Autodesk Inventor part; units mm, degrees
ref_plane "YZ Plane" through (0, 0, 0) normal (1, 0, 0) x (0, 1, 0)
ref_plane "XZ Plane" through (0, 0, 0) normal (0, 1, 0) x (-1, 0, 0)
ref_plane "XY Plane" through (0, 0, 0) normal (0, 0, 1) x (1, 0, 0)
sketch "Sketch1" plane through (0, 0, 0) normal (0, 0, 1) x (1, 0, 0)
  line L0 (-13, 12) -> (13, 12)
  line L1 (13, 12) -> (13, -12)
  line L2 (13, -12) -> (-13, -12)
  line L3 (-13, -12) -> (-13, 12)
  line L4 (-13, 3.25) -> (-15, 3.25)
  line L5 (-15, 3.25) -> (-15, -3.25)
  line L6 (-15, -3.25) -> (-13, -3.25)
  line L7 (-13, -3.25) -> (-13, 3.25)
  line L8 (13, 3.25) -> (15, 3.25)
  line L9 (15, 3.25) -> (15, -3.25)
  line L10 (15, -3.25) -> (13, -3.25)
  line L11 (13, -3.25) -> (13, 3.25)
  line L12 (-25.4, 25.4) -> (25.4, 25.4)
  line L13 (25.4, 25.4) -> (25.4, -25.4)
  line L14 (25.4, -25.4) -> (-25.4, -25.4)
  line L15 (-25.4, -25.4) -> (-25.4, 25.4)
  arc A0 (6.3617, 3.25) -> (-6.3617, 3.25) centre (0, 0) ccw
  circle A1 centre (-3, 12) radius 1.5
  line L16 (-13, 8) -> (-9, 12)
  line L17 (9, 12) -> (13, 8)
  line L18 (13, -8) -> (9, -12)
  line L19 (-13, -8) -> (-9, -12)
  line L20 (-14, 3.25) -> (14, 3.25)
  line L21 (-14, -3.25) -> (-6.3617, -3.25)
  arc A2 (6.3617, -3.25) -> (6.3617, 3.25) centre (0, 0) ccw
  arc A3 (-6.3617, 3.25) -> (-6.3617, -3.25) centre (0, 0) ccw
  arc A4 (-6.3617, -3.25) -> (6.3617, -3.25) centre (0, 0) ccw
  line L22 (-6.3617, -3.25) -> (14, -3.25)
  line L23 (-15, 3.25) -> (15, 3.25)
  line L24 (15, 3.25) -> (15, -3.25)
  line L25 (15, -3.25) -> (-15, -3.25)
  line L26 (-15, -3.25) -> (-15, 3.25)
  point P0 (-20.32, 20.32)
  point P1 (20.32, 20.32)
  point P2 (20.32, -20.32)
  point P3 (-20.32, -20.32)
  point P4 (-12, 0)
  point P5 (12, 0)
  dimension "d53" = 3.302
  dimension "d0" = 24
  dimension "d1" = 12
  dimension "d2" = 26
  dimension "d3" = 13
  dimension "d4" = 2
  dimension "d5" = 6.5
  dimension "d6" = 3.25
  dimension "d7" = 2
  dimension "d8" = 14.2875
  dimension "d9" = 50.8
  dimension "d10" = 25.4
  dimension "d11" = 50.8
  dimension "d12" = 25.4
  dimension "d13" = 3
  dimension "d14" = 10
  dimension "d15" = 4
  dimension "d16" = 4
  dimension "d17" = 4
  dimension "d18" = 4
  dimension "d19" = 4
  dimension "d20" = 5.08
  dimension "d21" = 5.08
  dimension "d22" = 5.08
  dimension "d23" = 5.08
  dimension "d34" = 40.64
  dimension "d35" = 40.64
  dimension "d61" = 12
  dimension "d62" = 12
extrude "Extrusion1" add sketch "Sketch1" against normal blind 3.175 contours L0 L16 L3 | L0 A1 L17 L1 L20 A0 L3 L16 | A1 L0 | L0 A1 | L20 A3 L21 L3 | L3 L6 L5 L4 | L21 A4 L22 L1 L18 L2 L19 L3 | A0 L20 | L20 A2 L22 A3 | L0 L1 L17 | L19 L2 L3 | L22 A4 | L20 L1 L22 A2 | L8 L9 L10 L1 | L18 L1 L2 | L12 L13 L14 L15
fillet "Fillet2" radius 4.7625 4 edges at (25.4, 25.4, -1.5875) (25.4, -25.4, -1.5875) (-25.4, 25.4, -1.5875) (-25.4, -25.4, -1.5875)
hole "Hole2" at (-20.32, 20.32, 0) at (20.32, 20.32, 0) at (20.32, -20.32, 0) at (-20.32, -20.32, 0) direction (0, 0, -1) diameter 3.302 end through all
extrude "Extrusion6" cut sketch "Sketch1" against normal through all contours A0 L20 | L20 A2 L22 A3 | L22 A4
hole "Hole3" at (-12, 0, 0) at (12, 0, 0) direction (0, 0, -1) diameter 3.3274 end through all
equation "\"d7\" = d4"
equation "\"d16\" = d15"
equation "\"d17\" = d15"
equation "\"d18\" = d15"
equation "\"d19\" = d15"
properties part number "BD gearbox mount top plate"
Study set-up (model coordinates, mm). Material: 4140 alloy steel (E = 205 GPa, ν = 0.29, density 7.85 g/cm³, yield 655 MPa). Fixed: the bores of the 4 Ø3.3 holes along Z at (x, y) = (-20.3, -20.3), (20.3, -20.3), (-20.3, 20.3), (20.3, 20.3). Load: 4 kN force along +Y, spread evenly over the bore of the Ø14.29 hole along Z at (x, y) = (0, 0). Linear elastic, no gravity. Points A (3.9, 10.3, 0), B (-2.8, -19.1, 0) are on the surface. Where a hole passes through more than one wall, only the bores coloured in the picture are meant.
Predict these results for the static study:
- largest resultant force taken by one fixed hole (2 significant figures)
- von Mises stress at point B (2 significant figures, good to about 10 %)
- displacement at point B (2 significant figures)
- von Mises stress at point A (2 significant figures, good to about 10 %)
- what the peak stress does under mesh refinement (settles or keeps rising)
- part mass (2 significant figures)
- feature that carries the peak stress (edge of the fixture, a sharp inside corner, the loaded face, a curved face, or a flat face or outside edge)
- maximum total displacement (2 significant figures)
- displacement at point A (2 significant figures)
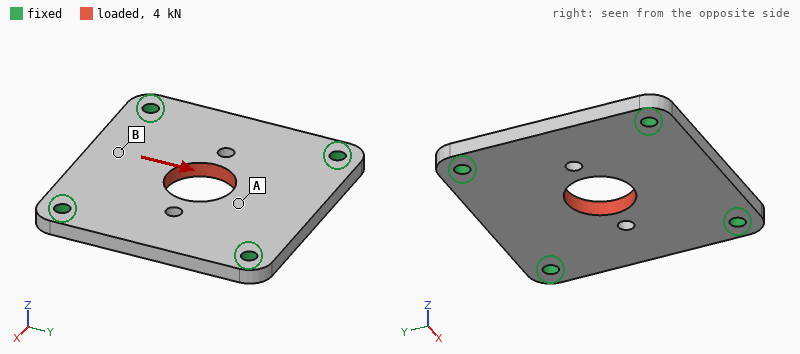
1.1 kN
10 MPa
3.4 µm
23 MPa
keeps rising
59 g
edge of the fixture
4.5 µm
3.8 µm
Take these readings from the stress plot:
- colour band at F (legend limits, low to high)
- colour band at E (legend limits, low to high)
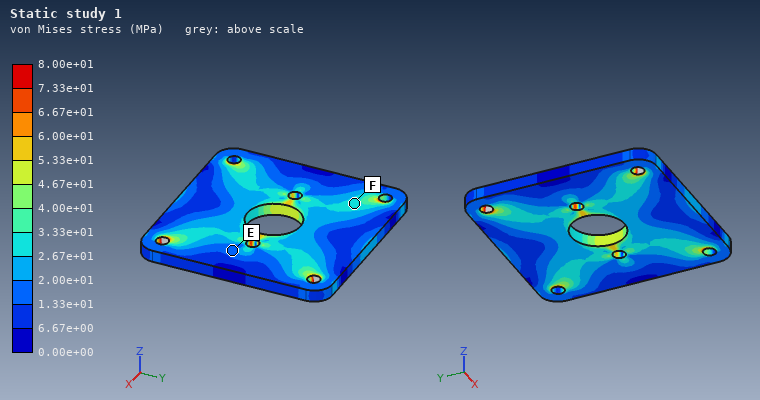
2.67e+01 to 3.33e+01 MPa
1.33e+01 to 2.00e+01 MPa
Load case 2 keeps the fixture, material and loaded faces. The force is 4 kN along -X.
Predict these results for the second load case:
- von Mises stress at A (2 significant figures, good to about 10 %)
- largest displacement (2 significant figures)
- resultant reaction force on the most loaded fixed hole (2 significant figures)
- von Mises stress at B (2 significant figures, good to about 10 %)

29 MPa
4.6 µm
1.1 kN
13 MPa
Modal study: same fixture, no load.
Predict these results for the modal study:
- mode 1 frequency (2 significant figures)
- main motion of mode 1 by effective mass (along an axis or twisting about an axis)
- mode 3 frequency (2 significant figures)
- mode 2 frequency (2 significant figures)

7000 Hz
along Z
11 kHz
11 kHz
